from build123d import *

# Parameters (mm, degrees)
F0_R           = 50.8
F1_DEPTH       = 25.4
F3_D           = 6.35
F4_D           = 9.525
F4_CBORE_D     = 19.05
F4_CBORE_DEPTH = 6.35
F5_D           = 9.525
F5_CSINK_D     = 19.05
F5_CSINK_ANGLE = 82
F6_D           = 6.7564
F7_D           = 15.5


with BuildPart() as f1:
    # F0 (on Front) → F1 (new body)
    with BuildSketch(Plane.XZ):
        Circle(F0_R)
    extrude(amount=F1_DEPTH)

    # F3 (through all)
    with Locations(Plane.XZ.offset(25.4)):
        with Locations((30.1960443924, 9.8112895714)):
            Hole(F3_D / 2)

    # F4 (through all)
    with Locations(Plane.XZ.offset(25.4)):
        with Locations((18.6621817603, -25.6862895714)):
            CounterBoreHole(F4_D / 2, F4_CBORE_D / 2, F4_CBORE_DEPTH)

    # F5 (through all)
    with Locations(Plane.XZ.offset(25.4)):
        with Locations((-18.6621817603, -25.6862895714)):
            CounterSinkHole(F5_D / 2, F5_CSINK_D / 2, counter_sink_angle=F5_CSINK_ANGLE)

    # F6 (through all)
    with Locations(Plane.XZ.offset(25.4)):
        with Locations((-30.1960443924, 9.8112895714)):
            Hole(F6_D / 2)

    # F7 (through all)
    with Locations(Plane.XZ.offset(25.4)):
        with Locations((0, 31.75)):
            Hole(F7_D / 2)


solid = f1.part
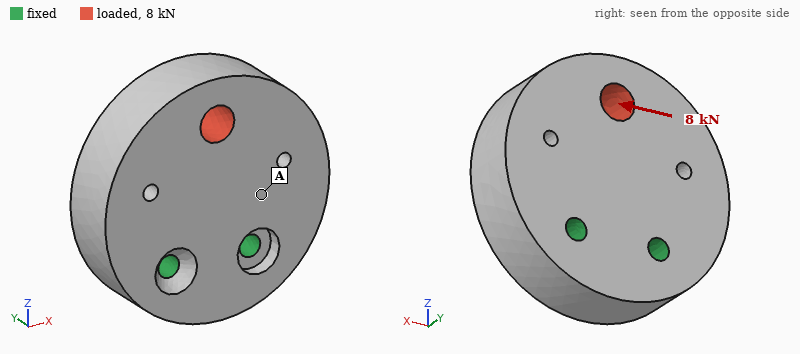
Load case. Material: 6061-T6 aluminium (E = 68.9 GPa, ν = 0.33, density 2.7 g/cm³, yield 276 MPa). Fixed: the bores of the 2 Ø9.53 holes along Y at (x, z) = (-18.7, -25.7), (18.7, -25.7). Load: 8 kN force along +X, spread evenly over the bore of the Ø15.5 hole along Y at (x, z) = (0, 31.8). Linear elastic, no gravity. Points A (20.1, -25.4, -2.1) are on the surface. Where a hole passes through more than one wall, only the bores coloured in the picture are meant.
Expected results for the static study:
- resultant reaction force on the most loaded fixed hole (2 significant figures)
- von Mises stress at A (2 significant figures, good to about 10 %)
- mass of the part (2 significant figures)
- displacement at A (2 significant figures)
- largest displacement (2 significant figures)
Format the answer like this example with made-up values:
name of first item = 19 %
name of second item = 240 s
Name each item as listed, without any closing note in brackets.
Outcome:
resultant reaction force on the most loaded fixed hole = 11 kN
von Mises stress at A = 8.2 MPa
mass of the part = 520 g
displacement at A = 11 µm
largest displacement = 31 µm
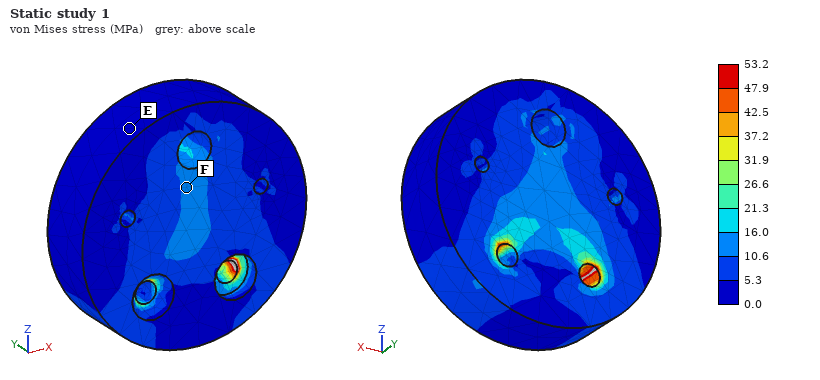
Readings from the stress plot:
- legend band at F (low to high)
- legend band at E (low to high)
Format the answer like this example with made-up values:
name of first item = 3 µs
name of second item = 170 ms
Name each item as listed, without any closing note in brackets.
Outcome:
legend band at F = 10.6 to 16.0 MPa
legend band at E = 0.0 to 5.3 MPa
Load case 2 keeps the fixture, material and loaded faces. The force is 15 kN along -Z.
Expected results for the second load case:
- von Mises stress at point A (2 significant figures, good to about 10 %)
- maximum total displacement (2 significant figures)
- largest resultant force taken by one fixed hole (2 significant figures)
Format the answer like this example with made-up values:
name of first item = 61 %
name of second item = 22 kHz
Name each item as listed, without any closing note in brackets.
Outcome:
von Mises stress at point A = 8.3 MPa
maximum total displacement = 17 µm
largest resultant force taken by one fixed hole = 7.6 kN
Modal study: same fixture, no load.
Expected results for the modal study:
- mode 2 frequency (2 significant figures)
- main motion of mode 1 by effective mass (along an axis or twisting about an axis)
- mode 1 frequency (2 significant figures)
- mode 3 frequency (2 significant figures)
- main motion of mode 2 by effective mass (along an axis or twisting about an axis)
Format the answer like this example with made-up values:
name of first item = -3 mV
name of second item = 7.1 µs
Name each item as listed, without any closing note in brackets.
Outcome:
mode 2 frequency = 5800 Hz
main motion of mode 1 by effective mass = along Y
mode 1 frequency = 3200 Hz
mode 3 frequency = 6100 Hz
main motion of mode 2 by effective mass = along X
